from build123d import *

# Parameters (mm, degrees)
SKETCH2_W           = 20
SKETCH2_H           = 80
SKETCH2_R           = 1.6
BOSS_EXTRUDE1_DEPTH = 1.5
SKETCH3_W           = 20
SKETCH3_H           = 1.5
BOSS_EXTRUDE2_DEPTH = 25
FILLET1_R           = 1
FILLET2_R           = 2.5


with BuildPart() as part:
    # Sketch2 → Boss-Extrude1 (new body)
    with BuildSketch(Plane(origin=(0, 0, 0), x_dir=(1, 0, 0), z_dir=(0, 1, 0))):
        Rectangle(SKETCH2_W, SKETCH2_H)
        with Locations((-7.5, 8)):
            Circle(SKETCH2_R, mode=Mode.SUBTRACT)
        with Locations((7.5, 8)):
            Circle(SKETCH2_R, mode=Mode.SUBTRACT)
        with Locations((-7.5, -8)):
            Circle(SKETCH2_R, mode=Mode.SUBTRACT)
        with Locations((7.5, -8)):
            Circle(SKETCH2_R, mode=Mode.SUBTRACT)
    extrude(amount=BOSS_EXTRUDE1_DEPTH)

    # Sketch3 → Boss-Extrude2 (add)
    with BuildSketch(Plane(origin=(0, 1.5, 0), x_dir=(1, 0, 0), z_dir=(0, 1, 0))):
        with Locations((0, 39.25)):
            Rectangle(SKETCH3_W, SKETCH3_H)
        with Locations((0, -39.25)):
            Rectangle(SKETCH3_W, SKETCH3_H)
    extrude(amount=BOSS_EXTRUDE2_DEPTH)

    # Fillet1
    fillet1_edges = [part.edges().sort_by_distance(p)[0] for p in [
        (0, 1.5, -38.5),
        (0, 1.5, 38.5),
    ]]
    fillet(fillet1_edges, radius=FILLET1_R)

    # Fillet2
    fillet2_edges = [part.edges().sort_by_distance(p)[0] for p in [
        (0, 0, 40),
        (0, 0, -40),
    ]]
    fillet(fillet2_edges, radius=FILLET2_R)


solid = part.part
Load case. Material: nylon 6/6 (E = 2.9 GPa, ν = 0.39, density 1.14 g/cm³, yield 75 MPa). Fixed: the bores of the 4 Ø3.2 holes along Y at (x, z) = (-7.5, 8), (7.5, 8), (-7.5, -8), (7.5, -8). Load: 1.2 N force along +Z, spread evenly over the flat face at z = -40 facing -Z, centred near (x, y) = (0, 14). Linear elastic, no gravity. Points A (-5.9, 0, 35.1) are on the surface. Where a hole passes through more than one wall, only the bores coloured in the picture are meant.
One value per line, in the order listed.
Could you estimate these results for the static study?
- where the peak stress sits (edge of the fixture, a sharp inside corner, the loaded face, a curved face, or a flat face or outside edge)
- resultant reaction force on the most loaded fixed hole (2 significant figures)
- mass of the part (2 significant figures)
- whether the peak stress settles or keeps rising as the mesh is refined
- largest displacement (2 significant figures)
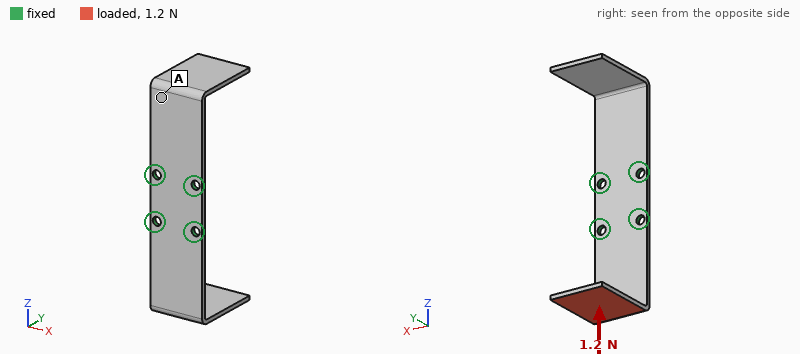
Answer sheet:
edge of the fixture
0.56 N
4.3 g
keeps rising
1.0 mm
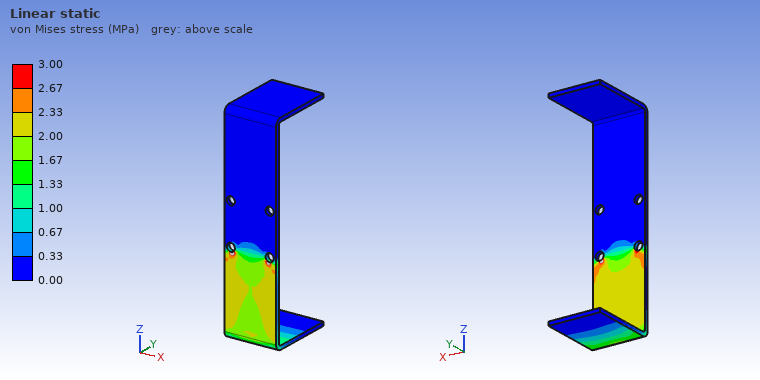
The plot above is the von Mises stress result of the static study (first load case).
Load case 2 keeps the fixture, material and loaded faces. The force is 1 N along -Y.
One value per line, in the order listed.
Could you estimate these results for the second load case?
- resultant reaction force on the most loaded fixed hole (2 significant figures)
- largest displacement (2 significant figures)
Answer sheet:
0.63 N
0.96 mm
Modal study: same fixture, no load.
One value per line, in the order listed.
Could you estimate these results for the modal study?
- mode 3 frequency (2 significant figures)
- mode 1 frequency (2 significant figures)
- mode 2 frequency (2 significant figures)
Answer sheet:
330 Hz
170 Hz
170 Hz
